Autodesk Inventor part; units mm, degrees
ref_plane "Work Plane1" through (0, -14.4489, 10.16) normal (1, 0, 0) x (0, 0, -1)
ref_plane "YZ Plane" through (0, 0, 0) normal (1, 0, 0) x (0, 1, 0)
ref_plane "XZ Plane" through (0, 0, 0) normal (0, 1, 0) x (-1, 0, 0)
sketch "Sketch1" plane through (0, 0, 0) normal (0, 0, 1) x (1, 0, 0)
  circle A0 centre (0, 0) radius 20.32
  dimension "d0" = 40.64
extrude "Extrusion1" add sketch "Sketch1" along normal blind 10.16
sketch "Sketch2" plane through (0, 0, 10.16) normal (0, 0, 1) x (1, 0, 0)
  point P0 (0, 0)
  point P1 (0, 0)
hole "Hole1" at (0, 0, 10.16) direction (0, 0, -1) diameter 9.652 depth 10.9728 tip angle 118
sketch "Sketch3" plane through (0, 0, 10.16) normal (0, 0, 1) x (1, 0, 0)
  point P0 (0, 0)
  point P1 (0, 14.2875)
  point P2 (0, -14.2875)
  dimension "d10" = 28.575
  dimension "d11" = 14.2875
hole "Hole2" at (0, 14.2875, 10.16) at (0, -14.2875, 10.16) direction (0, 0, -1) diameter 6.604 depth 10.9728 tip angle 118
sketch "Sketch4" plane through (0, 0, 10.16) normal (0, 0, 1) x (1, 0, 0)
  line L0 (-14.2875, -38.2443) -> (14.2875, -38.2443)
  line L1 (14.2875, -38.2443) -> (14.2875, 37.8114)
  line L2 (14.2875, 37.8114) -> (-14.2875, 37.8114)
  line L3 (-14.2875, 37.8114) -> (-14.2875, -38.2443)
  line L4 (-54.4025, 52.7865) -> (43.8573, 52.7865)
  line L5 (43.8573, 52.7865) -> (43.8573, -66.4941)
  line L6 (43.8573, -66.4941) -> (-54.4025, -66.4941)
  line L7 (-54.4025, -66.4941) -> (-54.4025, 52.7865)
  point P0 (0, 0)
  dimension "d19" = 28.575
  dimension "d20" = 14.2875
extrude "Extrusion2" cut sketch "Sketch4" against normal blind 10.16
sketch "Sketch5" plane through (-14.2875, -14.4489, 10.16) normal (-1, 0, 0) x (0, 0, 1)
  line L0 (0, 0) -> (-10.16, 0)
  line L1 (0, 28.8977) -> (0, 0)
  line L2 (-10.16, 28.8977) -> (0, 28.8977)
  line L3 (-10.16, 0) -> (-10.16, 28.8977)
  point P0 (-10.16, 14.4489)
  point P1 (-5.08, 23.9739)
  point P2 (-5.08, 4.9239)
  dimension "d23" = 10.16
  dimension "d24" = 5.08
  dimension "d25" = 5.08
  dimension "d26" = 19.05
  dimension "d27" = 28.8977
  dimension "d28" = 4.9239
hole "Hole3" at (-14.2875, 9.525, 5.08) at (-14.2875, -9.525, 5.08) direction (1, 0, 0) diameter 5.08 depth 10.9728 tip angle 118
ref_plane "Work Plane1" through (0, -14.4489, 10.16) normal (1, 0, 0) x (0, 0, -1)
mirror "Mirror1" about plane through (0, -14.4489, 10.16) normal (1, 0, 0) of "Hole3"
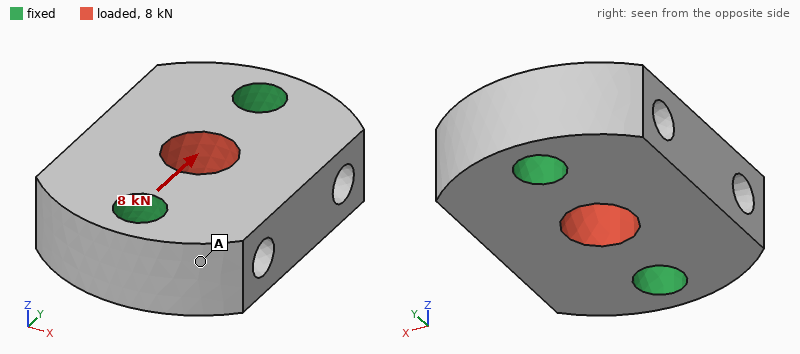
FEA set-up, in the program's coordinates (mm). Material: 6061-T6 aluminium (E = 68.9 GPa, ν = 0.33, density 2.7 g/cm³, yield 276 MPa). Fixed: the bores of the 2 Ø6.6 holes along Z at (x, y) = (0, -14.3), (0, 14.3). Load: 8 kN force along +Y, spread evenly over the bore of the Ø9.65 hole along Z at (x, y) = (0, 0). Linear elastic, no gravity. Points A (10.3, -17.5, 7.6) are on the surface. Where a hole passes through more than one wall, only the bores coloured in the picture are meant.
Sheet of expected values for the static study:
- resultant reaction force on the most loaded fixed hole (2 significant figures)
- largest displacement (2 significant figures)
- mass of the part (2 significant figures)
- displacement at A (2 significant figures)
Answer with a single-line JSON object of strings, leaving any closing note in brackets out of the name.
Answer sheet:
{"resultant reaction force on the most loaded fixed hole": "4.0 kN", "largest displacement": "6.1 µm", "mass of the part": "23 g", "displacement at A": "2.4 µm"}
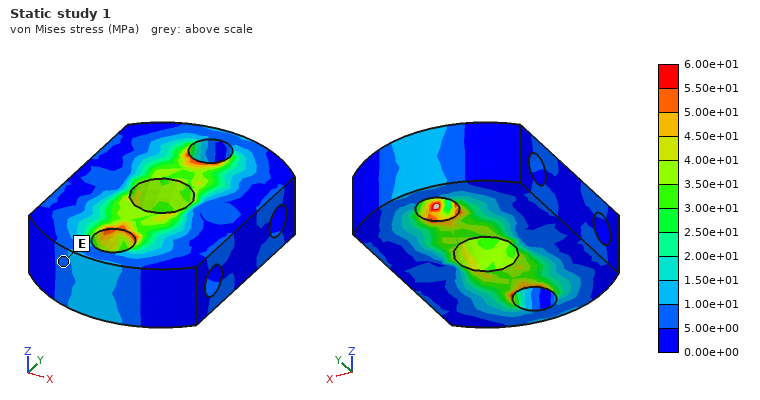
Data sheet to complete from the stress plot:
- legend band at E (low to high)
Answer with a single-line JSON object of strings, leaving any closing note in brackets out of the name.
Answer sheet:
{"legend band at E": "5.00e+00 to 1.00e+01 MPa"}
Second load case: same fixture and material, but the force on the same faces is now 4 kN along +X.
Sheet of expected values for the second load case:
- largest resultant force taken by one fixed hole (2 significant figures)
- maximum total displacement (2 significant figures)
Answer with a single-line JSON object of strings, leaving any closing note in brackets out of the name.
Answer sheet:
{"largest resultant force taken by one fixed hole": "2.0 kN", "maximum total displacement": "5.3 µm"}
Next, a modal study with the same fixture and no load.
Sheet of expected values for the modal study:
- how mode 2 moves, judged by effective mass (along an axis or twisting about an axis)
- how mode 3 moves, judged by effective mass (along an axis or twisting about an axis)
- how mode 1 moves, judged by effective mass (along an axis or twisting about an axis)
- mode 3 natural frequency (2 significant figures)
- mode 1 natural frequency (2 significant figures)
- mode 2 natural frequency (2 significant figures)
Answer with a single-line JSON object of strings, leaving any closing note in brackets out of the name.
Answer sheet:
{"how mode 2 moves, judged by effective mass": "along Z", "how mode 3 moves, judged by effective mass": "along X", "how mode 1 moves, judged by effective mass": "twisting about Y", "mode 3 natural frequency": "47 kHz", "mode 1 natural frequency": "27 kHz", "mode 2 natural frequency": "29 kHz"}
